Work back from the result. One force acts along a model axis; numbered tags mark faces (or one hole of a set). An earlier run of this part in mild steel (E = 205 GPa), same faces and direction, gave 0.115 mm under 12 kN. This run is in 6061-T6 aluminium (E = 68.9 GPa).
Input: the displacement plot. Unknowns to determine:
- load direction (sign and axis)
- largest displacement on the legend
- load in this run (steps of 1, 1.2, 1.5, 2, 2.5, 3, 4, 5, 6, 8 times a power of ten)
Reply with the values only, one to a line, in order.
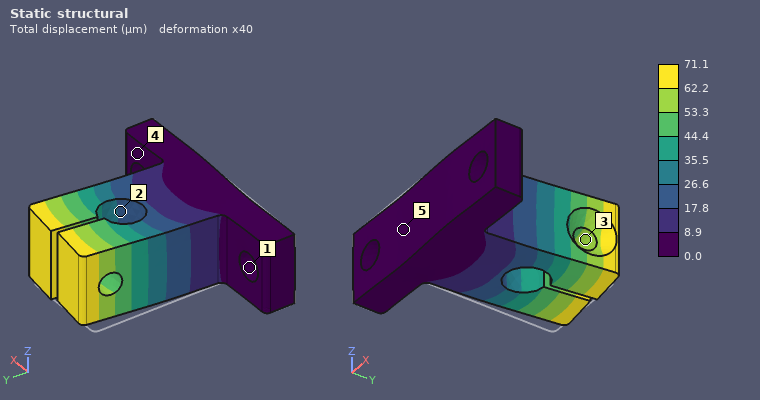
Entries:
+X
71.1 µm
2.5 kN
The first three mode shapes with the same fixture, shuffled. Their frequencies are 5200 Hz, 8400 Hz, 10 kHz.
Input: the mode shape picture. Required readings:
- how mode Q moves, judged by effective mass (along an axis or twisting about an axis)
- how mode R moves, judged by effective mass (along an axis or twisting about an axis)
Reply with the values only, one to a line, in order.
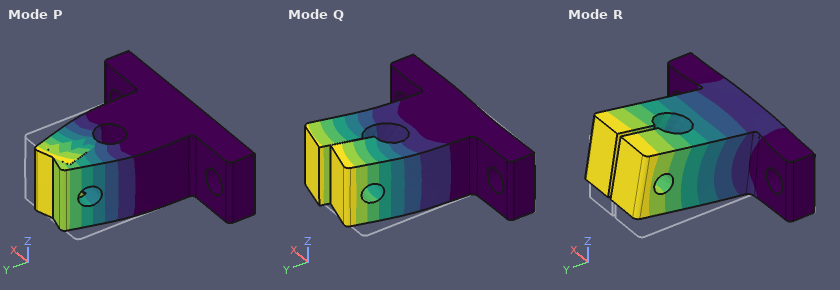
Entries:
along X
along Z
